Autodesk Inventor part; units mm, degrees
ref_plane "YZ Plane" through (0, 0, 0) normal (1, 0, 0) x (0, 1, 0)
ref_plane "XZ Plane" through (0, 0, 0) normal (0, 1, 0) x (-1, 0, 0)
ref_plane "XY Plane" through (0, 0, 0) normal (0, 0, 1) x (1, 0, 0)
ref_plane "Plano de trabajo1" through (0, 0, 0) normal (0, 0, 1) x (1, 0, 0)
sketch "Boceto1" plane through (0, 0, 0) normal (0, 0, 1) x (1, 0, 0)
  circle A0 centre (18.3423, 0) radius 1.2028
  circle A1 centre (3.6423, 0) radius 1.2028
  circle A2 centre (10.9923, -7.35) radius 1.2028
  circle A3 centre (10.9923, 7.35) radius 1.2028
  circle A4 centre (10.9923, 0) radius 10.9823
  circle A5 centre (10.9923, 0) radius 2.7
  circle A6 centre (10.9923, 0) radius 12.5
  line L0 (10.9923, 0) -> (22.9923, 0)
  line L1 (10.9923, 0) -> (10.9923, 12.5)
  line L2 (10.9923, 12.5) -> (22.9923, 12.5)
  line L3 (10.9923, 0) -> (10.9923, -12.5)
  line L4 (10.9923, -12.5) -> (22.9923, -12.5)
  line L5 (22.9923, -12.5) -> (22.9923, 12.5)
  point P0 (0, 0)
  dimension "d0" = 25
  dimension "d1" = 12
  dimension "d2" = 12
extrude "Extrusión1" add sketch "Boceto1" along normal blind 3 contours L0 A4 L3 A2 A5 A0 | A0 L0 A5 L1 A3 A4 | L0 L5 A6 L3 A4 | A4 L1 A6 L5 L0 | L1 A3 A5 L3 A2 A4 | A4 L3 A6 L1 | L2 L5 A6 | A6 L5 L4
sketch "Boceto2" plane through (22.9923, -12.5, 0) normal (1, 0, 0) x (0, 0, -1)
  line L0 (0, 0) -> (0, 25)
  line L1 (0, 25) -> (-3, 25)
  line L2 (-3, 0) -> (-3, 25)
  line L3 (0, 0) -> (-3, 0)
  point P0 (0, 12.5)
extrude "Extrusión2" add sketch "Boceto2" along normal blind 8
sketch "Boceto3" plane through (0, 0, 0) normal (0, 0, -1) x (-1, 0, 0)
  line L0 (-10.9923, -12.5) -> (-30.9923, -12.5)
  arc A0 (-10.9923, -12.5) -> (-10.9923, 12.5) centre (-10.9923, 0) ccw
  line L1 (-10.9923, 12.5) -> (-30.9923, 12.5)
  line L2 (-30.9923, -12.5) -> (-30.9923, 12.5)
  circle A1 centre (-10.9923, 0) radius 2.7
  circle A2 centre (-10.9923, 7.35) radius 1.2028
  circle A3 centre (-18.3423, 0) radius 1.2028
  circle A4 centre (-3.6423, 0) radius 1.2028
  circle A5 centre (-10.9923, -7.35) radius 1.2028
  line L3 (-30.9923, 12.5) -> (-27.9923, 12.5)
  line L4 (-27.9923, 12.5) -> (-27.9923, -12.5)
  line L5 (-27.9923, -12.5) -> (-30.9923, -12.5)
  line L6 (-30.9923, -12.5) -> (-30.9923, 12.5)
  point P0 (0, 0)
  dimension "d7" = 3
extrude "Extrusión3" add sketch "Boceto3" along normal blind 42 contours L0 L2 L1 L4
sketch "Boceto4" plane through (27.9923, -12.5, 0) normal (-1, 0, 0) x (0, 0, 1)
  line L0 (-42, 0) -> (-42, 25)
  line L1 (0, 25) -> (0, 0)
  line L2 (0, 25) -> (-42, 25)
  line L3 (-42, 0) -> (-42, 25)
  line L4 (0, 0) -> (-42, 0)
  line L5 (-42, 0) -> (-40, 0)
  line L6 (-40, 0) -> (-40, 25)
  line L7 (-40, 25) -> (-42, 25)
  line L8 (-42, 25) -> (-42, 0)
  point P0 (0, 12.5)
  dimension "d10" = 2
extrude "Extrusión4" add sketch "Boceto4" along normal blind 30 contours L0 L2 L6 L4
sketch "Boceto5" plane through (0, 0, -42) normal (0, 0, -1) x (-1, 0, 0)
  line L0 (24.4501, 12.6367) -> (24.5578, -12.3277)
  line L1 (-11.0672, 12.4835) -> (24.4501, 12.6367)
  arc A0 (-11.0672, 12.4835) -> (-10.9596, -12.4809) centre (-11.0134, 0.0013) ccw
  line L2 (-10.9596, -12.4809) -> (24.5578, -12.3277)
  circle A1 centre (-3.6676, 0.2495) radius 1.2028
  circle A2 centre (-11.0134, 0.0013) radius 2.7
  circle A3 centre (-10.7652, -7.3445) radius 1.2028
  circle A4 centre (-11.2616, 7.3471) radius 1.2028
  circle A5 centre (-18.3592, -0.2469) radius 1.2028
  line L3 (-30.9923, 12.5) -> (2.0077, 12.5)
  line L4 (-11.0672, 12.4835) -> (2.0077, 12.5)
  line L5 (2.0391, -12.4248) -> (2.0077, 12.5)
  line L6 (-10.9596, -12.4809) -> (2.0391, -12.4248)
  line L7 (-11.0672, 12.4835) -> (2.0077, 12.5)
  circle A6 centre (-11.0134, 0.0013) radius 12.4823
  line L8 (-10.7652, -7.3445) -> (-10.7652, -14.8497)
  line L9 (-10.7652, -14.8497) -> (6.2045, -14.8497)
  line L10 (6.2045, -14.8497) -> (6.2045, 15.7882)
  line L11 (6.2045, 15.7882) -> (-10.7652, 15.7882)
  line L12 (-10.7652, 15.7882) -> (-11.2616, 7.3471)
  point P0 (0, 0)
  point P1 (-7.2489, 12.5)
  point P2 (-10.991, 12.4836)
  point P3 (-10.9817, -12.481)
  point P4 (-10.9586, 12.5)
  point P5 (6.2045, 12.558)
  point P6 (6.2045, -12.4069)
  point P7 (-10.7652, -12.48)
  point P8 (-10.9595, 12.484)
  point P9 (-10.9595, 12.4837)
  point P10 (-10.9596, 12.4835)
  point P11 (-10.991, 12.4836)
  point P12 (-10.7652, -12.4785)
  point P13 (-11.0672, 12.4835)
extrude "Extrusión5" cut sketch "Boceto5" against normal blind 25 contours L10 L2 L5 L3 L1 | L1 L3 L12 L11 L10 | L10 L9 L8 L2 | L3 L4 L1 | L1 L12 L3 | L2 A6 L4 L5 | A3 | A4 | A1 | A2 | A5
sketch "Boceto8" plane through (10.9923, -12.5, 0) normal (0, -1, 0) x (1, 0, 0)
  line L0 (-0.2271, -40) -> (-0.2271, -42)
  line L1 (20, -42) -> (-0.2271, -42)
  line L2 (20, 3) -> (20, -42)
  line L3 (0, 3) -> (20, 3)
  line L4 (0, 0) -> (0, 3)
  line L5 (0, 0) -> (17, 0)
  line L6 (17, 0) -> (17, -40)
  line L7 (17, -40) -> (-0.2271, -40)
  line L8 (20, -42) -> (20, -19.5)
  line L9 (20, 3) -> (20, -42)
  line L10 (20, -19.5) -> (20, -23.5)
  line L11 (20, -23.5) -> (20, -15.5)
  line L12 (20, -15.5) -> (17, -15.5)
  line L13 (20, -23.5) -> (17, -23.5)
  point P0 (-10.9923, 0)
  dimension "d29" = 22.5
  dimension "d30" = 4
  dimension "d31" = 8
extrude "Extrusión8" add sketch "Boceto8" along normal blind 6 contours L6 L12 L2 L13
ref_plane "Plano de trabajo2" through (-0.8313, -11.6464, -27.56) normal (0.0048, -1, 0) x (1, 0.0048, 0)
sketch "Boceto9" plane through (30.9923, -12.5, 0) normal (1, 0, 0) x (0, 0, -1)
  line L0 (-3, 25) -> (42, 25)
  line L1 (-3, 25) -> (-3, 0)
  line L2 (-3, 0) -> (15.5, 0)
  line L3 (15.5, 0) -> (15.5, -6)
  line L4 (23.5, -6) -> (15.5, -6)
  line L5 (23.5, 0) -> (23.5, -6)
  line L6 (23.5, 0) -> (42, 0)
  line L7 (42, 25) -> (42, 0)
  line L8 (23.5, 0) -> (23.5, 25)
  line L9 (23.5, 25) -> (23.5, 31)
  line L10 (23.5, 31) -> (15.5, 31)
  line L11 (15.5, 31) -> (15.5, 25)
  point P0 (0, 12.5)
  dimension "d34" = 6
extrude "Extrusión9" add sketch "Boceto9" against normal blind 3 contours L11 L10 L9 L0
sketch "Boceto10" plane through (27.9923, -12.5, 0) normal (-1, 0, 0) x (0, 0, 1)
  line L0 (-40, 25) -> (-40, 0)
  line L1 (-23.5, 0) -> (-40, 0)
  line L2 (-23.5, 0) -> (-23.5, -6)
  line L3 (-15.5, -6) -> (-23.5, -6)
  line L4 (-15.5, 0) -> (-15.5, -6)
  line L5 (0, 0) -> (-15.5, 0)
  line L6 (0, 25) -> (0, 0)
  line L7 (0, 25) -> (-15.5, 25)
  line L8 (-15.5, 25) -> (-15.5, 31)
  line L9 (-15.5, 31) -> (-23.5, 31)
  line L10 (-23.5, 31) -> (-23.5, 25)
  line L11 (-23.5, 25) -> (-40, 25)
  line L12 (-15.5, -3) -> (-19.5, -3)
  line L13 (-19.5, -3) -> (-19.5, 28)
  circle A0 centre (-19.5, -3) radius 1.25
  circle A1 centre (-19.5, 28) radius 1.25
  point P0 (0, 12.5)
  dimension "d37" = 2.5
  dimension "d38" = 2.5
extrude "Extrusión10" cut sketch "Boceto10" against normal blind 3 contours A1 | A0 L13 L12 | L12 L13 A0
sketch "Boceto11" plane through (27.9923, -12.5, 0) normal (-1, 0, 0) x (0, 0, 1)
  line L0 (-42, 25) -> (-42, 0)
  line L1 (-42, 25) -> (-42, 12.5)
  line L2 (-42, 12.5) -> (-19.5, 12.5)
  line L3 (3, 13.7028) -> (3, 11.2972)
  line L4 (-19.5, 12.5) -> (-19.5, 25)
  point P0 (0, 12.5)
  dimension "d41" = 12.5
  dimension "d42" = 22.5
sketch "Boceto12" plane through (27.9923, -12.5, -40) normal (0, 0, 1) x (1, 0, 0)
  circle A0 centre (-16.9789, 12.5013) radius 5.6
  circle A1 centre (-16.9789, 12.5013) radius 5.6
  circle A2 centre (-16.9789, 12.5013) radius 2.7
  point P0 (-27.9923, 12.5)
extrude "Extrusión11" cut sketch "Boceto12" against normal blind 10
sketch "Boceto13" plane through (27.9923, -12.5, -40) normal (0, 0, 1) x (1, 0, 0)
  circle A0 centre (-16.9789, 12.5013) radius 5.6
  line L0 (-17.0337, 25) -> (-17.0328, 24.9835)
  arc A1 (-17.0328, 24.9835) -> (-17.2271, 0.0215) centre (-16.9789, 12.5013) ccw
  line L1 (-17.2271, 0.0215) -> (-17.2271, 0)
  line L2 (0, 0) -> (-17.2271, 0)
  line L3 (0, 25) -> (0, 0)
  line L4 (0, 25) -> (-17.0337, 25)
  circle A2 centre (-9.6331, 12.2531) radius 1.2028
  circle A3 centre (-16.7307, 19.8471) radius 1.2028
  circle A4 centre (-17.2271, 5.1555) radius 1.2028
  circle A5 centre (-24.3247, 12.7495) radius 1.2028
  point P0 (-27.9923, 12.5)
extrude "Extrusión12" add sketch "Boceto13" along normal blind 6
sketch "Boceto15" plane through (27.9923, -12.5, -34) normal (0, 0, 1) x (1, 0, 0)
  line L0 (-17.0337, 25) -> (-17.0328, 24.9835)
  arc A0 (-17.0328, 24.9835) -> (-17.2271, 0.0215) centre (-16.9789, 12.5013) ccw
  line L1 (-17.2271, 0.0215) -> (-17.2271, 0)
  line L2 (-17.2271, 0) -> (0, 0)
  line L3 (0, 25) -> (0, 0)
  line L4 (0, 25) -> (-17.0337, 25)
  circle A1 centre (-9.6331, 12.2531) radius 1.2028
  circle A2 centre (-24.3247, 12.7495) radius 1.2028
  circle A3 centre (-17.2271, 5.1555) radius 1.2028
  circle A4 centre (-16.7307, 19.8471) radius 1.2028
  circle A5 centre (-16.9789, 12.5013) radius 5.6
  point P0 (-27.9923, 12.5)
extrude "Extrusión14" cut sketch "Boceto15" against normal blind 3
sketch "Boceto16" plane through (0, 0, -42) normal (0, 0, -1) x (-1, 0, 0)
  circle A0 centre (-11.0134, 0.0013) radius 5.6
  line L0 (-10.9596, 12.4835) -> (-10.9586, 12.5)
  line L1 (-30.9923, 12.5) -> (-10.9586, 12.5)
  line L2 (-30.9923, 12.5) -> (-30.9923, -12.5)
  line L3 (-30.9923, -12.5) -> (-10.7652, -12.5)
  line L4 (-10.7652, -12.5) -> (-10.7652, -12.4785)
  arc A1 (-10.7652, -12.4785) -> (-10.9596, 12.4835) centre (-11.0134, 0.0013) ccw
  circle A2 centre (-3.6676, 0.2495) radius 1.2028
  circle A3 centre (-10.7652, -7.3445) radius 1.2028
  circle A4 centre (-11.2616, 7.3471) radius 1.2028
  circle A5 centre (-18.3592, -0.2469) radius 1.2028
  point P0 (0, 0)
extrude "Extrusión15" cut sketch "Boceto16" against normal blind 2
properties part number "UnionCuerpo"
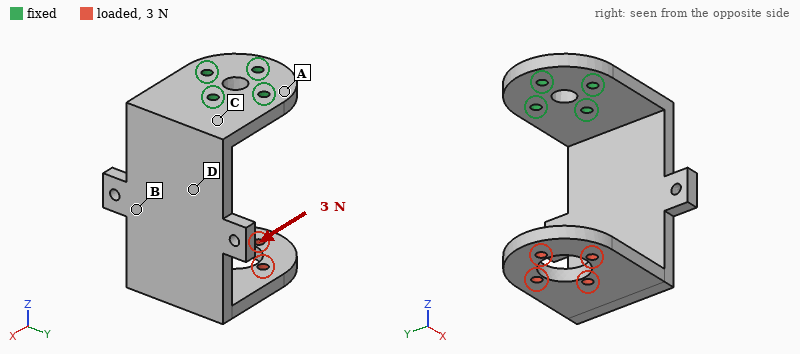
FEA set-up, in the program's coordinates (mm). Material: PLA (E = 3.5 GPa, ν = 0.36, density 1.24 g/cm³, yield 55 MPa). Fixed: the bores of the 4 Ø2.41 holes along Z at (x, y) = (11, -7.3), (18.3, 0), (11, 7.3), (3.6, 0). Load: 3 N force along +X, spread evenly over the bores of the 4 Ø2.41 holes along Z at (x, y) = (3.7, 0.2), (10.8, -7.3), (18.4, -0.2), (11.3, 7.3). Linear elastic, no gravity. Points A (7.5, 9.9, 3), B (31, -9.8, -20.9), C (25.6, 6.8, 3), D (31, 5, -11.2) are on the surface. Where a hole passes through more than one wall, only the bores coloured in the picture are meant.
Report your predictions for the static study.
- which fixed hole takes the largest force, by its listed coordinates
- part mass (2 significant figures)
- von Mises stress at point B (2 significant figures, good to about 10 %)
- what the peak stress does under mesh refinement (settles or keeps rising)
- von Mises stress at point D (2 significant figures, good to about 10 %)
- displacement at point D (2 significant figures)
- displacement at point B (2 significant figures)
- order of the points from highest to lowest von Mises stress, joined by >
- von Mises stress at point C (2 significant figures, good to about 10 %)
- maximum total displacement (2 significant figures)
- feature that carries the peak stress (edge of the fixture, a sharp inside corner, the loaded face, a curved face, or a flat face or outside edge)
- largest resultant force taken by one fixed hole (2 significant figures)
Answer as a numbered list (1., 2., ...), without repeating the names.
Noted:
1. (18.3, 0)
2. 8.7 g
3. 1.2 MPa
4. keeps rising
5. 2.0 MPa
6. 0.13 mm
7. 0.26 mm
8. C > D > B > A
9. 2.8 MPa
10. 0.77 mm
11. edge of the fixture
12. 9.2 N
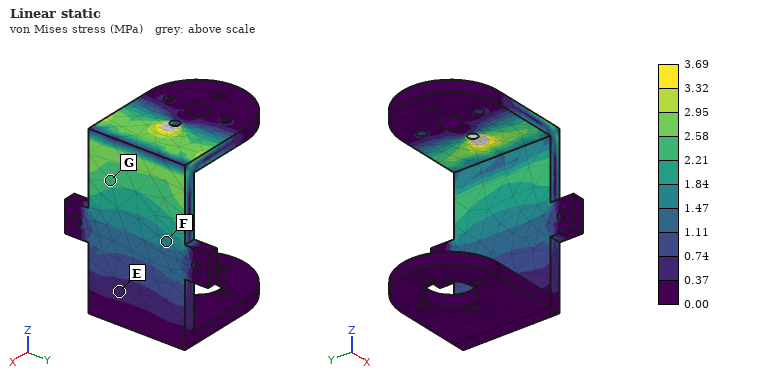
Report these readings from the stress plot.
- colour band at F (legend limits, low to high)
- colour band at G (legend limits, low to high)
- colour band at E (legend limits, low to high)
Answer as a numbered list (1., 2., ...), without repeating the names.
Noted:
1. 1.47 to 1.84 MPa
2. 2.21 to 2.58 MPa
3. 0.37 to 0.74 MPa
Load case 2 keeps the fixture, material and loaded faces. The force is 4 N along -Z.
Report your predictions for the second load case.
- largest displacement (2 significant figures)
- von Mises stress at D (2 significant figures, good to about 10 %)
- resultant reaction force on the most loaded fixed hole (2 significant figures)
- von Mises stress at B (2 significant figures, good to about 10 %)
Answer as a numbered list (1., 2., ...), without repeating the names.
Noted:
1. 0.71 mm
2. 1.8 MPa
3. 1.8 N
4. 1.7 MPa
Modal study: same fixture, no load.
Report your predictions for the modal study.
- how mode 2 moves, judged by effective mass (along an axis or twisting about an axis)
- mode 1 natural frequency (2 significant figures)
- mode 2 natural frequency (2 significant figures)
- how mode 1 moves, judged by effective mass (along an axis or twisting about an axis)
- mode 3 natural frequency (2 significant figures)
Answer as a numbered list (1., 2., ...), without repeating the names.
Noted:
1. along Y
2. 190 Hz
3. 310 Hz
4. along X
5. 640 Hz
